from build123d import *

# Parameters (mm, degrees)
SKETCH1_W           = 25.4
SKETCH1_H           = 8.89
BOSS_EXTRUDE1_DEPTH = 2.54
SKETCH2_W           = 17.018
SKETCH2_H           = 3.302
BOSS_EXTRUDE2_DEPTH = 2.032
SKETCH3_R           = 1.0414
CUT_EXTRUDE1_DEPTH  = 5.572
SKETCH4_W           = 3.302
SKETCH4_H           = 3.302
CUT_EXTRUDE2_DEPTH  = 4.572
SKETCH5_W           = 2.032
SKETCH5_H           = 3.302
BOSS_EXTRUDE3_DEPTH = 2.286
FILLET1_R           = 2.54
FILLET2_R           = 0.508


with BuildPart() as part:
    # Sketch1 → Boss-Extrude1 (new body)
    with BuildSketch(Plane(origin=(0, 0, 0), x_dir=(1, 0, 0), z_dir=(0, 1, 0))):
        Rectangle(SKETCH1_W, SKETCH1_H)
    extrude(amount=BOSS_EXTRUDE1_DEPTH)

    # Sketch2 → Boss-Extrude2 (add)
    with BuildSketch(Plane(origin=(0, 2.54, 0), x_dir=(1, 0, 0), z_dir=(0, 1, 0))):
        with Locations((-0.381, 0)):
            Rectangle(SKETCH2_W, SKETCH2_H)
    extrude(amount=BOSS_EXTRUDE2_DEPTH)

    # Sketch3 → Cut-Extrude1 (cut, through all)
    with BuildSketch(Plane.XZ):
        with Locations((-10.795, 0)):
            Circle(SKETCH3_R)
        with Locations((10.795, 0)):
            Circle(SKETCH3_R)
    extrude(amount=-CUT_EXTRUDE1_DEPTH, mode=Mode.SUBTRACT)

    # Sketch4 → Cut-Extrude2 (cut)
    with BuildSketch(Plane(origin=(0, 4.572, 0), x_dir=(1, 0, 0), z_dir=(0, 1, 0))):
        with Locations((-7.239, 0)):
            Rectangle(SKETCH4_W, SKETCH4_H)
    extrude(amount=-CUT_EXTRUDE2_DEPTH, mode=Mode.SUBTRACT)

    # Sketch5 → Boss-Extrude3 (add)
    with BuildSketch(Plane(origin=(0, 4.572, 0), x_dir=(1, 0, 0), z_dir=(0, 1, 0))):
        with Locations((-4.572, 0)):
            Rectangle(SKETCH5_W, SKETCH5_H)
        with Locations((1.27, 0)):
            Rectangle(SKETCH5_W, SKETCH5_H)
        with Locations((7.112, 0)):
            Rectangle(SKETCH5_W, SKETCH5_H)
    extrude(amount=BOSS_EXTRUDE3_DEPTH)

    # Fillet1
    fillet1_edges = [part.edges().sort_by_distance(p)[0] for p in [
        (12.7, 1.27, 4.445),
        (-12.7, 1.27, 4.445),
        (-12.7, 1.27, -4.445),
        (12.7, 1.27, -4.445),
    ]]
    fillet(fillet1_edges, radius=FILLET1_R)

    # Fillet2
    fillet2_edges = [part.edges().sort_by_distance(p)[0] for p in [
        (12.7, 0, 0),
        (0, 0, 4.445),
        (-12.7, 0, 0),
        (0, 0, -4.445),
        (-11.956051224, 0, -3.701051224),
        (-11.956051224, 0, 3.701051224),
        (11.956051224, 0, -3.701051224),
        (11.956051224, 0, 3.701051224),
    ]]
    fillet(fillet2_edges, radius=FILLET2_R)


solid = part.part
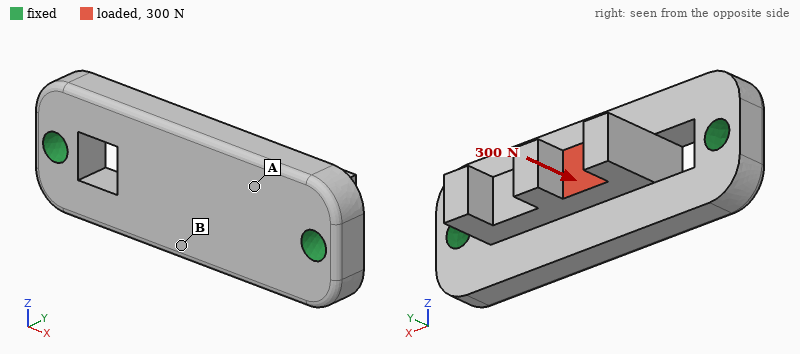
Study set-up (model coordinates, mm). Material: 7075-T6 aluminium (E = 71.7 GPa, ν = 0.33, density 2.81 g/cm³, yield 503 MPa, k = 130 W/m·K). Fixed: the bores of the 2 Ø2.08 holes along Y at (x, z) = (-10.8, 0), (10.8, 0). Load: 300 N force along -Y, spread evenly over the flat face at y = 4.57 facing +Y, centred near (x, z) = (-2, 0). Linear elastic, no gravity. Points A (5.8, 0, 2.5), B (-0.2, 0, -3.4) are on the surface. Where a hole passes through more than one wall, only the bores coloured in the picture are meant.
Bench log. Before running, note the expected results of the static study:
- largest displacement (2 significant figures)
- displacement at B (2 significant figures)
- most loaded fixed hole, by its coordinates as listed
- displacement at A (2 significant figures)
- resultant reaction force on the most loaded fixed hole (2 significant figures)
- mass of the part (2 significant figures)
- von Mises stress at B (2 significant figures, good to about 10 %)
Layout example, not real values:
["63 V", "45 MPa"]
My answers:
["17 µm", "15 µm", "(-10.8, 0)", "6.8 µm", "180 N", "1.8 g", "36 MPa"]
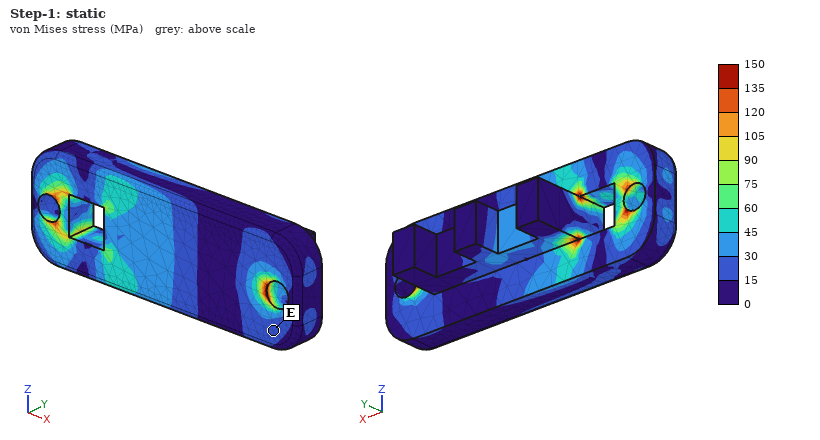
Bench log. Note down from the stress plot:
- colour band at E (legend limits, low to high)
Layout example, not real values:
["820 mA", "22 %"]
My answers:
["15 to 30 MPa"]
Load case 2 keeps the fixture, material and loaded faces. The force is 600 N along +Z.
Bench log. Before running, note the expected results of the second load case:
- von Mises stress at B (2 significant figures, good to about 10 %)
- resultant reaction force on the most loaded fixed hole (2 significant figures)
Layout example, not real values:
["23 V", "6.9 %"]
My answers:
["72 MPa", "320 N"]
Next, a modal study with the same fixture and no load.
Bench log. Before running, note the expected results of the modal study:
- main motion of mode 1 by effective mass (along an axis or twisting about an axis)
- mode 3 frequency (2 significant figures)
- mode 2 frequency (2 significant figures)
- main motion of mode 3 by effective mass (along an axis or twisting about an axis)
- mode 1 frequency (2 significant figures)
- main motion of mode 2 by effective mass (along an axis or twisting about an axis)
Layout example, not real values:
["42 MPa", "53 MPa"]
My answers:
["along Y", "36 kHz", "27 kHz", "along Z", "23 kHz", "along Z"]
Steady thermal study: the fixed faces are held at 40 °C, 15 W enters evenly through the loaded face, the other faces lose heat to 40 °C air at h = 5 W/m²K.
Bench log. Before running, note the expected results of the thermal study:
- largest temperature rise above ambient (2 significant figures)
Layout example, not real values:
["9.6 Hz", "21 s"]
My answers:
["45 K"]
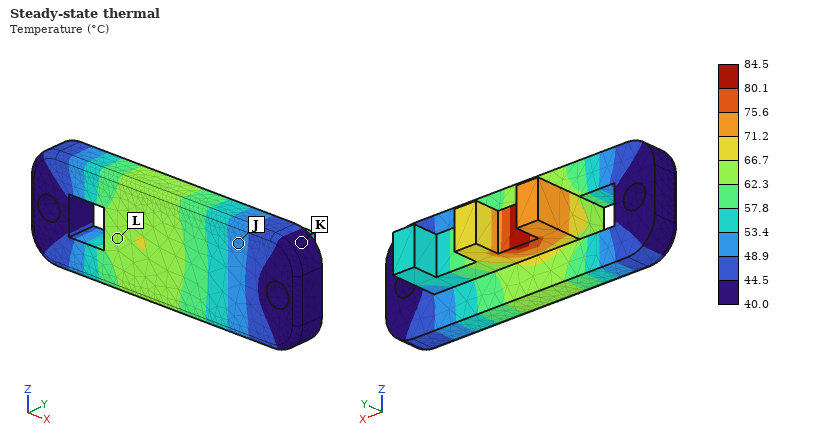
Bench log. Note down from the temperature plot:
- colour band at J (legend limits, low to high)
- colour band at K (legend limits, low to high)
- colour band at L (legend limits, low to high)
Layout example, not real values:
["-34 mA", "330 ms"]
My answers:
["48.9 to 53.4 °C", "40.0 to 44.5 °C", "62.3 to 66.7 °C"]
